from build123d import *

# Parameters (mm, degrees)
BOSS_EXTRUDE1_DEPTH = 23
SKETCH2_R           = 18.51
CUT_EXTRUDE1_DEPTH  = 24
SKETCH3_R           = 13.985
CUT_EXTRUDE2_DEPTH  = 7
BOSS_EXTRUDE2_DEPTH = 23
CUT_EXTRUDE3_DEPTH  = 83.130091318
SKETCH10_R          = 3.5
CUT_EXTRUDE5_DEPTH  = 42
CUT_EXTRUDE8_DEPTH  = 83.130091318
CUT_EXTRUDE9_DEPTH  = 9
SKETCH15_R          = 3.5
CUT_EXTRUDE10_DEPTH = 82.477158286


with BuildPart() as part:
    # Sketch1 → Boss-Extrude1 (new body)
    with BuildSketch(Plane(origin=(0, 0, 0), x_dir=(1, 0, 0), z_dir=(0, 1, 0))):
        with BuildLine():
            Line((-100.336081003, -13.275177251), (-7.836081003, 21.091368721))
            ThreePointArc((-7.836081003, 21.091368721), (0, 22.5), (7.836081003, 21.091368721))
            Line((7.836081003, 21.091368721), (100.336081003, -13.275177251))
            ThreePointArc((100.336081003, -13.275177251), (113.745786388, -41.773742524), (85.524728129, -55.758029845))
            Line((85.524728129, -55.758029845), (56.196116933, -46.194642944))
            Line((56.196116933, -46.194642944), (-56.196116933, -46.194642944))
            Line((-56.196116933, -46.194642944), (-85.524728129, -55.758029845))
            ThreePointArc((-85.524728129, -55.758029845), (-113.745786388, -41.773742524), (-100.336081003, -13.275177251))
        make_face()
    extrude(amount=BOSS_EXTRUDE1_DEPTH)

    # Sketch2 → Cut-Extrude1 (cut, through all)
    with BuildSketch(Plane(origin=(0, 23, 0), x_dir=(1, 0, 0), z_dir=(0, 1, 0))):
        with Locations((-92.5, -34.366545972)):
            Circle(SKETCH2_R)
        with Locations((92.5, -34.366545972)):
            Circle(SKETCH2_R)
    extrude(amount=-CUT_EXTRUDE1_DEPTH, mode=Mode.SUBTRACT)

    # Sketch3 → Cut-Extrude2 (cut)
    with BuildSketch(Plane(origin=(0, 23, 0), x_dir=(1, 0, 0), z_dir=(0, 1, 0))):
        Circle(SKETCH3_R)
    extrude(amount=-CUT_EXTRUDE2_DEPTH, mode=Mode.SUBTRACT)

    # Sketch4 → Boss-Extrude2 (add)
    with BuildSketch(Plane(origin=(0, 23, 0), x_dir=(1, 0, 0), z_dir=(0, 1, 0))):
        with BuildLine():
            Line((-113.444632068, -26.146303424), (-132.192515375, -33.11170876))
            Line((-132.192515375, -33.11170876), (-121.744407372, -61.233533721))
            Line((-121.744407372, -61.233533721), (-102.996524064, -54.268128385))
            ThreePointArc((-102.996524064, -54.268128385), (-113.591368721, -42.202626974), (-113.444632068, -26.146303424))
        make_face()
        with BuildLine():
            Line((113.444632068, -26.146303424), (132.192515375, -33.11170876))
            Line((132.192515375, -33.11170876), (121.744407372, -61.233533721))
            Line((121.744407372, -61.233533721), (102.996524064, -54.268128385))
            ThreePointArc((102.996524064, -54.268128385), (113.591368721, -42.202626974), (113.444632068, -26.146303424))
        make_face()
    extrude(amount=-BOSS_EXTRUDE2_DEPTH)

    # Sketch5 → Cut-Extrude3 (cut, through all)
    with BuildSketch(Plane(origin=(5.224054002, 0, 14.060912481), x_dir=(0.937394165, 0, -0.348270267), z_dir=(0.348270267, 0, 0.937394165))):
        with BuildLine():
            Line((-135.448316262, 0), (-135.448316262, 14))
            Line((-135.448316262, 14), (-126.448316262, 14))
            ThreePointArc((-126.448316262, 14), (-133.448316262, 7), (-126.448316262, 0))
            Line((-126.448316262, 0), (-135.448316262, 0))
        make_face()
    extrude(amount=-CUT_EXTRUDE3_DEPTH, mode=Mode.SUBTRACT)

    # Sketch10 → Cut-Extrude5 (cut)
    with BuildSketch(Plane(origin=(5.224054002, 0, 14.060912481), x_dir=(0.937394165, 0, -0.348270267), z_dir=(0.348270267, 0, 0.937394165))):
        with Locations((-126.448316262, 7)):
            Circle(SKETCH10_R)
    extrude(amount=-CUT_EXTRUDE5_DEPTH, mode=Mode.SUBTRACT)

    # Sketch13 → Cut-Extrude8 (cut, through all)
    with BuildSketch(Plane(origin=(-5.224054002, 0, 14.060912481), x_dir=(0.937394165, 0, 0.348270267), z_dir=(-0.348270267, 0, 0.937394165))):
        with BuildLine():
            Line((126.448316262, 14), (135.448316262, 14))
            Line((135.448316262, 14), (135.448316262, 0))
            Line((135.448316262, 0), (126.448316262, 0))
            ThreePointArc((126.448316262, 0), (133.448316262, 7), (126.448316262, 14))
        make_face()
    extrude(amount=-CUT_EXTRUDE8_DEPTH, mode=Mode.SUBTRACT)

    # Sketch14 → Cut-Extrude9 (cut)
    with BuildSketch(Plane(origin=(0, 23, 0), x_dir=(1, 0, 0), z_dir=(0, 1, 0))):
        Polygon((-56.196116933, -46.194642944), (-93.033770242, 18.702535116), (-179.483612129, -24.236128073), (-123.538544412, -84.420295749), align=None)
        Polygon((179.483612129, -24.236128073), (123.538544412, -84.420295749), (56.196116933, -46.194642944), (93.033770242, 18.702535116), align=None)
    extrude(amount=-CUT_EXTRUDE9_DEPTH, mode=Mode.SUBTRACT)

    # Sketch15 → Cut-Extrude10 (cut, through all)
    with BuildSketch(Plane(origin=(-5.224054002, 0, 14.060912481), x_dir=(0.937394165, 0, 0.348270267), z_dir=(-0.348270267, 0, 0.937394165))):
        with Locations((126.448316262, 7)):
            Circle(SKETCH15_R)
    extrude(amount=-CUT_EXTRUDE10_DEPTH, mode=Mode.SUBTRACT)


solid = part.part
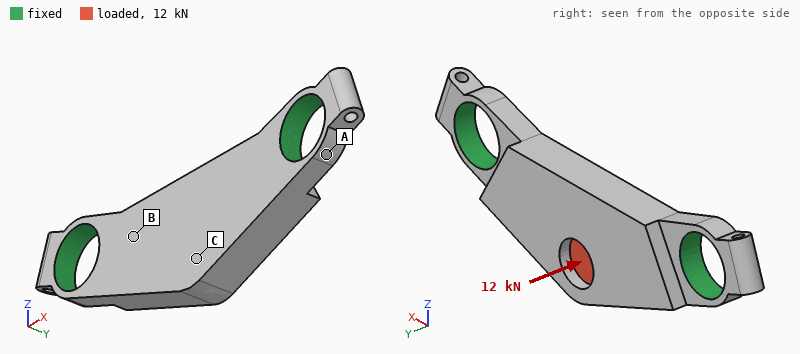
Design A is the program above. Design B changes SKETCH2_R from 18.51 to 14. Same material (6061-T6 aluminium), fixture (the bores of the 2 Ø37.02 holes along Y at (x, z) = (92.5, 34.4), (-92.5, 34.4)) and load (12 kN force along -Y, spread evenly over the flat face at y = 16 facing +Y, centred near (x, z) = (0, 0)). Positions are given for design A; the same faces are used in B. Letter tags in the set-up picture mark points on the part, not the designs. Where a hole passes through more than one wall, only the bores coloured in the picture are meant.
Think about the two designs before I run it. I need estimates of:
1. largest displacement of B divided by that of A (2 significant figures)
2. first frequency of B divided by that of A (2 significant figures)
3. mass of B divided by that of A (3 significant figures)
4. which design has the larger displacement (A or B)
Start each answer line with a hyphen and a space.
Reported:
- 1.2
- 0.88
- 1.06
- B
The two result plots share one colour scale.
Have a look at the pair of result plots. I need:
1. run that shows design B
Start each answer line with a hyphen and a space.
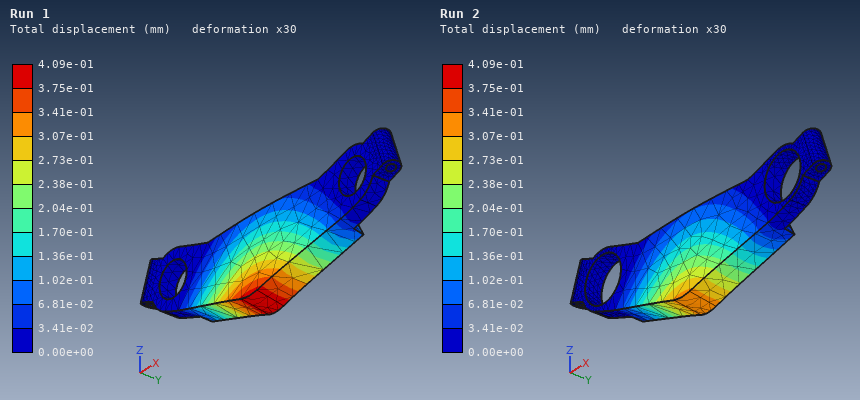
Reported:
- Run 1
